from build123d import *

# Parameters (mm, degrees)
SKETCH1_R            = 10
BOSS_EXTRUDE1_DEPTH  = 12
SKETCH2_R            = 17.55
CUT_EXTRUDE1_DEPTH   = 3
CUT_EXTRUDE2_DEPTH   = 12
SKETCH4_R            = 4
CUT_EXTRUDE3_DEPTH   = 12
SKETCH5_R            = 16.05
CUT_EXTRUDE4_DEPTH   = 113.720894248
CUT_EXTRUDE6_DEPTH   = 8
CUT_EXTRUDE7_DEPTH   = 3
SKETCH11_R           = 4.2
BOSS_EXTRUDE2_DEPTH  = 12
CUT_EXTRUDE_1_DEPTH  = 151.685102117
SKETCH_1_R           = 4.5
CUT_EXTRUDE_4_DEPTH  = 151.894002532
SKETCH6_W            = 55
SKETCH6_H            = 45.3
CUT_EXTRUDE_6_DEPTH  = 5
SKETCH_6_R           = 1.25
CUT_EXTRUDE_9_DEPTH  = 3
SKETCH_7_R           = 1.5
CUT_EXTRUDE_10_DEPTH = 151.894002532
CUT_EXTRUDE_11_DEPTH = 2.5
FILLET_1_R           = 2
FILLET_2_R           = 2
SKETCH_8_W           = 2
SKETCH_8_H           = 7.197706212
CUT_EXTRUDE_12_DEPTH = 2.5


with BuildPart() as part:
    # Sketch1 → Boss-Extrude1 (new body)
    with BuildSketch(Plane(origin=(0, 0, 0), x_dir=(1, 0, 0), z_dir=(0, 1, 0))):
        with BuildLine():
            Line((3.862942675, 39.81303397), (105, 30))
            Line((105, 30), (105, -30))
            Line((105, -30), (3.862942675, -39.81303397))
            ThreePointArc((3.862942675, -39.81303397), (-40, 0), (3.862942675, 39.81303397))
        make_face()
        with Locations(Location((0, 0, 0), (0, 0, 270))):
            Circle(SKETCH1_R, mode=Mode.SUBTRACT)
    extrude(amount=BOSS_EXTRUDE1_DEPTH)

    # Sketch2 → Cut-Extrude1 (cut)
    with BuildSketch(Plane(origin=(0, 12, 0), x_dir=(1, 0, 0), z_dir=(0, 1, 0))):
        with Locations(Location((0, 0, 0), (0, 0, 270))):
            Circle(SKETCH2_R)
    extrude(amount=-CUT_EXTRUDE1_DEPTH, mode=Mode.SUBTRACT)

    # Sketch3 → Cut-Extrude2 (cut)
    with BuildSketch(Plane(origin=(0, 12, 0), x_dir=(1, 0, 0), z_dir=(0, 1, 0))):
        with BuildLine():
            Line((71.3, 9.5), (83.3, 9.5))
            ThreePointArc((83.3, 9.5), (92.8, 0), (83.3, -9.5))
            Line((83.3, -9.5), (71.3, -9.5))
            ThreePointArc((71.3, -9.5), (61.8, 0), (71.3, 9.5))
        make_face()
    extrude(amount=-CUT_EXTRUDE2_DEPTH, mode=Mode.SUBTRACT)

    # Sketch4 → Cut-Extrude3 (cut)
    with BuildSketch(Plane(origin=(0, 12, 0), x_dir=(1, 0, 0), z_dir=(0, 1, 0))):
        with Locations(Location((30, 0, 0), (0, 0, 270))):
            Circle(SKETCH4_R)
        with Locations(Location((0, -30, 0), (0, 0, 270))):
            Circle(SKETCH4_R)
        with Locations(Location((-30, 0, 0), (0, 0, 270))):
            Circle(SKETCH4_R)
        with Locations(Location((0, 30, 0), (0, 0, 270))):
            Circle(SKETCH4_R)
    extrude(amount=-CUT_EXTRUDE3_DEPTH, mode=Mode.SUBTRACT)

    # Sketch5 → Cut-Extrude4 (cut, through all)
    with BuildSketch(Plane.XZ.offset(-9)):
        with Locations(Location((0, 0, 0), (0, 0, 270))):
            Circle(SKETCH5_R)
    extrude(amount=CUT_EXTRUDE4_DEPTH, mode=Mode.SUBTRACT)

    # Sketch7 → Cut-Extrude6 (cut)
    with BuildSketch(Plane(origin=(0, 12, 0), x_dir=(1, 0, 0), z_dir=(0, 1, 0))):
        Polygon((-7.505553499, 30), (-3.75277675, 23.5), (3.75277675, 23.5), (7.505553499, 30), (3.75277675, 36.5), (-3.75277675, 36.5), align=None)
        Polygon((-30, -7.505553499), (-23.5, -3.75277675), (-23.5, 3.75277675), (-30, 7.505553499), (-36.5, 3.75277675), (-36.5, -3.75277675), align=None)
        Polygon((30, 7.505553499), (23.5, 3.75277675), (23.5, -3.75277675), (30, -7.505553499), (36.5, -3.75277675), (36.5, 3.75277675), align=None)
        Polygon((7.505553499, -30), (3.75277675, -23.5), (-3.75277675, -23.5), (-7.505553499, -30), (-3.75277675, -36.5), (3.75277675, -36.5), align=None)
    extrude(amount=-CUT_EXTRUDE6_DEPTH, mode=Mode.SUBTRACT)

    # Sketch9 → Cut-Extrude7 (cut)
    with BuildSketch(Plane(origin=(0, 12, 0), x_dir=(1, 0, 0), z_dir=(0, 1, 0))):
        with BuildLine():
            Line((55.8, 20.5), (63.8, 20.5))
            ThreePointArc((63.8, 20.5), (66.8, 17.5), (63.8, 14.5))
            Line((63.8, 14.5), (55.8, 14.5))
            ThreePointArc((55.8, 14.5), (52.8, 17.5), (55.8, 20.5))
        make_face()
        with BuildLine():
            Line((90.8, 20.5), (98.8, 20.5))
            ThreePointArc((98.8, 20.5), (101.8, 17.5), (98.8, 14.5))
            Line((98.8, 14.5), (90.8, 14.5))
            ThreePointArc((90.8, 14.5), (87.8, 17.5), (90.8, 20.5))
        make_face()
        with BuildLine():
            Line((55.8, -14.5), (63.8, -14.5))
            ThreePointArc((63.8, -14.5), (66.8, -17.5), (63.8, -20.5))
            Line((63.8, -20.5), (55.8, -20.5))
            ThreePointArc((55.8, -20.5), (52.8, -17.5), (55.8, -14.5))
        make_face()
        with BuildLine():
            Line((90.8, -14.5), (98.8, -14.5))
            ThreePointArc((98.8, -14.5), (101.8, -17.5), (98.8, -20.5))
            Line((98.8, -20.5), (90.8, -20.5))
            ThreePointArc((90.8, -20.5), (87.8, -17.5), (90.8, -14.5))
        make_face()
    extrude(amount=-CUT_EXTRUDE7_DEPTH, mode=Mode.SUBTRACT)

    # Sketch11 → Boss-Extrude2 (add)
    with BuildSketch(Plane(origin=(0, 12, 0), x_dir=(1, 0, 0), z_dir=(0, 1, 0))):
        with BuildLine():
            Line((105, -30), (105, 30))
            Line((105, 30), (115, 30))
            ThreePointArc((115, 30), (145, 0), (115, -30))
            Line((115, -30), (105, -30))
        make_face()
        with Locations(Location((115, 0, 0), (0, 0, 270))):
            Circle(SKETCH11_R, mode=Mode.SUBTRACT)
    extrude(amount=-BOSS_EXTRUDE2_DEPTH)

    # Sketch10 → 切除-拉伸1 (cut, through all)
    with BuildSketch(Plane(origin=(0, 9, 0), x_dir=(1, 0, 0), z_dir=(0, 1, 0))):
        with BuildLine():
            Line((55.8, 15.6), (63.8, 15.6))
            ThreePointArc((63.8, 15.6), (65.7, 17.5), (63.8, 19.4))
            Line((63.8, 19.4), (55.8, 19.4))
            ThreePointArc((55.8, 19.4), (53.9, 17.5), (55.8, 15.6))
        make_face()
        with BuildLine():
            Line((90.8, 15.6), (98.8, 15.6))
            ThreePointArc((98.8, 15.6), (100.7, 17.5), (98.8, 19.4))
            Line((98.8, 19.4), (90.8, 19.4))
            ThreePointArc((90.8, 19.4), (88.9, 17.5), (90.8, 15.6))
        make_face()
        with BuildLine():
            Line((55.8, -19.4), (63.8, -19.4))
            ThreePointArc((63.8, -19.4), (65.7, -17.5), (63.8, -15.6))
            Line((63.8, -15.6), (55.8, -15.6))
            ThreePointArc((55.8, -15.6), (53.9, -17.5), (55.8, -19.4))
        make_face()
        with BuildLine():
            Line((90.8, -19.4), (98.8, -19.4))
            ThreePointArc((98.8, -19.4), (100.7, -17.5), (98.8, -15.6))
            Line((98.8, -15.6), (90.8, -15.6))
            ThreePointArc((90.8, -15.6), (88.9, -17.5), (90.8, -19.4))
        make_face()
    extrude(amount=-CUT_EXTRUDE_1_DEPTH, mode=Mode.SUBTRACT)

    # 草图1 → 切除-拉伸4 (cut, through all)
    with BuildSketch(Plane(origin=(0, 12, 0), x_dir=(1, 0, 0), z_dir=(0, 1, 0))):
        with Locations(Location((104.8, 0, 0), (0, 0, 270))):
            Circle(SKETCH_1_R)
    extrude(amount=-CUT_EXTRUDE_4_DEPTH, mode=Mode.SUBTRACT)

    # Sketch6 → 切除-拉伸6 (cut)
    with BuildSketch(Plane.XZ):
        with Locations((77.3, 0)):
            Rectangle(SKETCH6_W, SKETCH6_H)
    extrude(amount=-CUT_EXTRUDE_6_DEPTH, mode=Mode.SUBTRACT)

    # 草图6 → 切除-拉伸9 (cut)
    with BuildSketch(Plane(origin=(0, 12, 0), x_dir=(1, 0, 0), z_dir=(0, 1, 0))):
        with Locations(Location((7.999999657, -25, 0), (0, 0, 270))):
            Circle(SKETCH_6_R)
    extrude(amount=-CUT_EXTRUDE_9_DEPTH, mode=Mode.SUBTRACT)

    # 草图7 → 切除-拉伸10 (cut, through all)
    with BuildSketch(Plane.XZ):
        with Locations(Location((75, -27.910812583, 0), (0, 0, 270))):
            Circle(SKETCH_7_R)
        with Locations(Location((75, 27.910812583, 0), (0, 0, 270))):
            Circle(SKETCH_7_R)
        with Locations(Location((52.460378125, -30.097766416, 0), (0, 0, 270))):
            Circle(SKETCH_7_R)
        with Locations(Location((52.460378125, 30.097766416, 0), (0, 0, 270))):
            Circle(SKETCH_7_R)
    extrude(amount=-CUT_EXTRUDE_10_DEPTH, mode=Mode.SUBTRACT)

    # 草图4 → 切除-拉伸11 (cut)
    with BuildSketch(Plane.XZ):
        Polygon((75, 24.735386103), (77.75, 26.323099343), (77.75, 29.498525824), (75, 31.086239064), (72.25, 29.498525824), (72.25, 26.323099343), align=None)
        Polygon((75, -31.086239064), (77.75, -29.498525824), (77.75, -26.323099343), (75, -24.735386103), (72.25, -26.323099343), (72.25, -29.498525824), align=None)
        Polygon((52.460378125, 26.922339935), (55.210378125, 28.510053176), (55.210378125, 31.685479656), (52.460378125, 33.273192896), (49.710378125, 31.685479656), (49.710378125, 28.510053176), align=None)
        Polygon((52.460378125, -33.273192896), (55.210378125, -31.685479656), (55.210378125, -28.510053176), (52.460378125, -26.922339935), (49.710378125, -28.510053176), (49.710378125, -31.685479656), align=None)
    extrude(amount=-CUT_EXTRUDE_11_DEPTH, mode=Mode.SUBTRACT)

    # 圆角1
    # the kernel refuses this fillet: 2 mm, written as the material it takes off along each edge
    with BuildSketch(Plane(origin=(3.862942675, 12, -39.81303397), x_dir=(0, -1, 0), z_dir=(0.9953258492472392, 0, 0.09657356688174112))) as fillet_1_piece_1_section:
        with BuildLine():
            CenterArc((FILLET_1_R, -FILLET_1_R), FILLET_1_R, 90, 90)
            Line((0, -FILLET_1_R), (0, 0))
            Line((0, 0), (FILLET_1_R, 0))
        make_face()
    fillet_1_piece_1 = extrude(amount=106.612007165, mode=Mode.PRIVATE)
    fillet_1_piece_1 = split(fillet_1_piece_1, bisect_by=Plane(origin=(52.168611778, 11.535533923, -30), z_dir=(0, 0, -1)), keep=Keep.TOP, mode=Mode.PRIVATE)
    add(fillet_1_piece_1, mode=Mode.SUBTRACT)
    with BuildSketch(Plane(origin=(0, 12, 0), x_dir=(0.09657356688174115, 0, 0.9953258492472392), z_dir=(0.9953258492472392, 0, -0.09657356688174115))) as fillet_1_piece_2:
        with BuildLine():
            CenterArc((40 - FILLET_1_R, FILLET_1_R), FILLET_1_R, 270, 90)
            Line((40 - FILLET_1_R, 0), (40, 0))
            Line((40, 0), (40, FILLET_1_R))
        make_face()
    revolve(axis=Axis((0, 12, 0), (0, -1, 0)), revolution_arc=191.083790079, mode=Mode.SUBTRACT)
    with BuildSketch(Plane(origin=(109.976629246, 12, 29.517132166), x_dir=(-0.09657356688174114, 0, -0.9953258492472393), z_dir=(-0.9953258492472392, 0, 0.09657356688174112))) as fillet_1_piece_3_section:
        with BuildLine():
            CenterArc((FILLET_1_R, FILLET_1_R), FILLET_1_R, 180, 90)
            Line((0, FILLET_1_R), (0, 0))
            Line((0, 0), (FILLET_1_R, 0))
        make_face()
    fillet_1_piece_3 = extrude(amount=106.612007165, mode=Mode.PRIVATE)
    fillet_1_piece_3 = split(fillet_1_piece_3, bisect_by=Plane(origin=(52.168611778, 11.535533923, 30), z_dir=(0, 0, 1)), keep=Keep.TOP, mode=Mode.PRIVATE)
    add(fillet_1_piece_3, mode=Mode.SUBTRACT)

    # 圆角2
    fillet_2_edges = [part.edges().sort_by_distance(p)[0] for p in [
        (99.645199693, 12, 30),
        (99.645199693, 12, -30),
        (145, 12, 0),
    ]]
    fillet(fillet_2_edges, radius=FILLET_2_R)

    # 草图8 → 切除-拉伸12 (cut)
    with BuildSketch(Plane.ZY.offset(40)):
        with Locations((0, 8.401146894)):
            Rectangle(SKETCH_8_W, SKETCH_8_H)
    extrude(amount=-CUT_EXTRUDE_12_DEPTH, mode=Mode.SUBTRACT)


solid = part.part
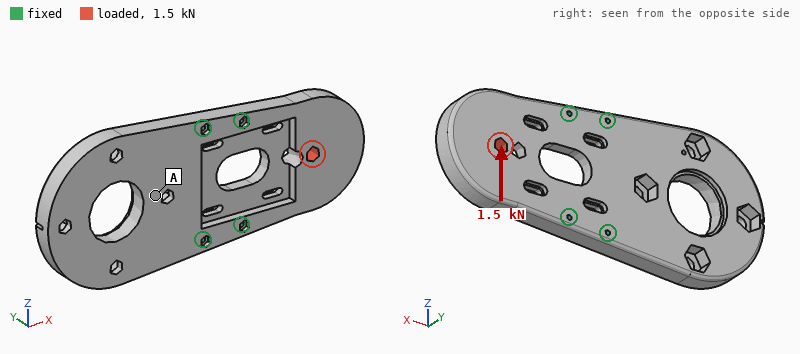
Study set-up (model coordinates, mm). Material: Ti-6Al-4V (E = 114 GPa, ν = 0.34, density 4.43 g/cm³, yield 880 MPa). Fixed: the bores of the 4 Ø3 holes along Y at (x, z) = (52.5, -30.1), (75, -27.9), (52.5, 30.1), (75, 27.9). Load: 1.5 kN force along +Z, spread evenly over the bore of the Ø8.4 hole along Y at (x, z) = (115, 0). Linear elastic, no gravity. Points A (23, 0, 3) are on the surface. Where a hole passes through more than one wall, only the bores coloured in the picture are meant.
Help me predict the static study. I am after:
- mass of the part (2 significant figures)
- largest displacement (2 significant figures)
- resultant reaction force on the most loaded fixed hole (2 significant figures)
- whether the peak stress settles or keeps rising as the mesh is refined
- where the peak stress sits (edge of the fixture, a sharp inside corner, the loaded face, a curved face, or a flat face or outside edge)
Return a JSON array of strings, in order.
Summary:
["480 g", "10 µm", "1.2 kN", "keeps rising", "edge of the fixture"]
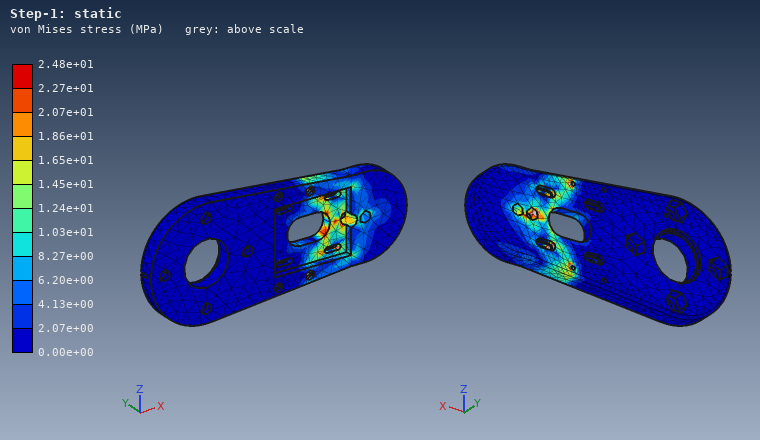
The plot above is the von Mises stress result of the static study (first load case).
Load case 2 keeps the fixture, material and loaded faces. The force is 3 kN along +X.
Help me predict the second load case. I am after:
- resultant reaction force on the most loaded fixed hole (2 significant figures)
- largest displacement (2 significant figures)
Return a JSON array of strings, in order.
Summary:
["1.2 kN", "20 µm"]
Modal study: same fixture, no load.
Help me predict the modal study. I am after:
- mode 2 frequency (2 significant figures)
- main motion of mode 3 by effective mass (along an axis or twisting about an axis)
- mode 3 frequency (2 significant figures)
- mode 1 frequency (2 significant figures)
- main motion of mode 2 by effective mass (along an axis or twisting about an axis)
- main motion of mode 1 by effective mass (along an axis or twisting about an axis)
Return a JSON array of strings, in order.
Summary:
["1400 Hz", "twisting about X", "3000 Hz", "1000 Hz", "along Y", "along Y"]
